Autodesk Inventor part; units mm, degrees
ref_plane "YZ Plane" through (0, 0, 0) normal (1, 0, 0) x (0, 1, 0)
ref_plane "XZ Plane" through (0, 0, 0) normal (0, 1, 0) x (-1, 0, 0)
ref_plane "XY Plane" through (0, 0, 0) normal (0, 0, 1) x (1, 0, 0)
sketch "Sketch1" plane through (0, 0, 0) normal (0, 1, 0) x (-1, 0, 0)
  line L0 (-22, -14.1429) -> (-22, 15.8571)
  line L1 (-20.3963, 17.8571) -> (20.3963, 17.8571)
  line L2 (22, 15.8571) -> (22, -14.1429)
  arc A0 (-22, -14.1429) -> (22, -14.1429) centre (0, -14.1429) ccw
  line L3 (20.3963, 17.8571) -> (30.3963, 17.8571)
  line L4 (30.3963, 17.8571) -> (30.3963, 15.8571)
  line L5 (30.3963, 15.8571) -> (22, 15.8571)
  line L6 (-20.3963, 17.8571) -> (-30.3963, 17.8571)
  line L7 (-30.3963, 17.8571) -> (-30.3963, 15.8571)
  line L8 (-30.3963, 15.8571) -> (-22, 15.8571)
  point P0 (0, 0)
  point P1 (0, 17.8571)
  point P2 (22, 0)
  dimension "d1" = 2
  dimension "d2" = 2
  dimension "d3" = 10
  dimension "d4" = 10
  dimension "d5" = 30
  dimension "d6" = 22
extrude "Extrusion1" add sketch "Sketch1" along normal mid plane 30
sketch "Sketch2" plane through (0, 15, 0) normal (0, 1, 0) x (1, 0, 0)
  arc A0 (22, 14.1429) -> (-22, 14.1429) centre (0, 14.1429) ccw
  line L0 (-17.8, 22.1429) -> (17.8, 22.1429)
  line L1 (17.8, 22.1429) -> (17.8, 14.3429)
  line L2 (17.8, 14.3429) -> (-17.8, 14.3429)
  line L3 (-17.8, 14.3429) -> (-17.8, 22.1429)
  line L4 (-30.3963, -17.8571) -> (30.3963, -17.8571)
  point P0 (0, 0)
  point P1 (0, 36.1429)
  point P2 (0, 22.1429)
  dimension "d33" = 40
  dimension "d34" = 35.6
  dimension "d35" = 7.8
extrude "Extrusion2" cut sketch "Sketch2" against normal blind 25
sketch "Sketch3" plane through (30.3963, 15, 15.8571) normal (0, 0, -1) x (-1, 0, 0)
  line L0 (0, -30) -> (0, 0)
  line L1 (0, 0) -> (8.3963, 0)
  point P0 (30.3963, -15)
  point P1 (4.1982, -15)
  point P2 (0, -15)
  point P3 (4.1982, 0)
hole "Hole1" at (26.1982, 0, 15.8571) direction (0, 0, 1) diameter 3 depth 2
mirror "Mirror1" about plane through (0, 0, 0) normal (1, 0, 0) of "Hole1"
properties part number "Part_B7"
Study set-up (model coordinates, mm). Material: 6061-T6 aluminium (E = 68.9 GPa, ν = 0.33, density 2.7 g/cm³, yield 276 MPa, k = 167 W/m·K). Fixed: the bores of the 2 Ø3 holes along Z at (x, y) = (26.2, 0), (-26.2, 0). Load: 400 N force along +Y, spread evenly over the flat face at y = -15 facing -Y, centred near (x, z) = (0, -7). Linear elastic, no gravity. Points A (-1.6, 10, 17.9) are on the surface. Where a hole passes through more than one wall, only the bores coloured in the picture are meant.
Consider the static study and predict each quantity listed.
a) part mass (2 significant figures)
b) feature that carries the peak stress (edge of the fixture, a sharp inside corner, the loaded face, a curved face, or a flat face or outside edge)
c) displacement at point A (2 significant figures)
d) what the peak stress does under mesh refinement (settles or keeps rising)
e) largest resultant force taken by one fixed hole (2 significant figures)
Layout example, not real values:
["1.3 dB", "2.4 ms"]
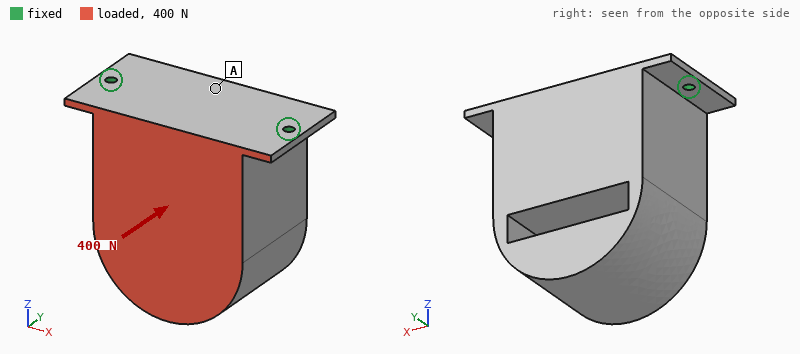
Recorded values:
["160 g", "edge of the fixture", "0.12 mm", "keeps rising", "200 N"]
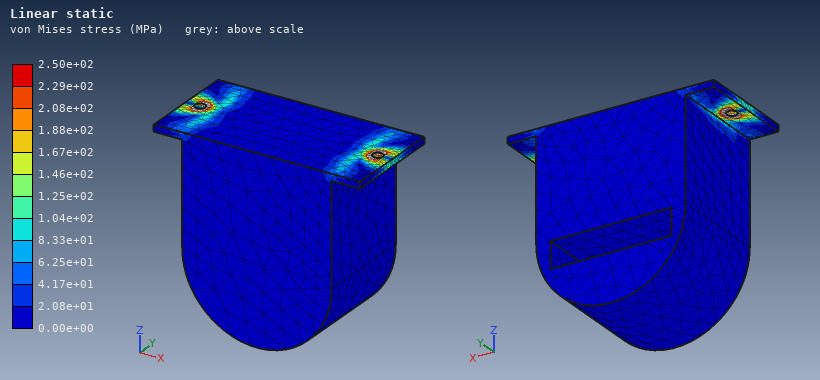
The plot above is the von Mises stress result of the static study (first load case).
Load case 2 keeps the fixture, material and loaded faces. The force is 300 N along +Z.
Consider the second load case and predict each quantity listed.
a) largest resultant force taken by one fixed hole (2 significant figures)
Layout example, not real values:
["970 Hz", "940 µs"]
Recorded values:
["170 N"]
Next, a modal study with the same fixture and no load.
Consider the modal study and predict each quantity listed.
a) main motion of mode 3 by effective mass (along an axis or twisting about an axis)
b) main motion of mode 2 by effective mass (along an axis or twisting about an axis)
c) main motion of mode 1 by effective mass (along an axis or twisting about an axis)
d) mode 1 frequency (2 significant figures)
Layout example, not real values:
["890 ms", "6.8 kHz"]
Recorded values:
["along Z", "along X", "along Y", "390 Hz"]
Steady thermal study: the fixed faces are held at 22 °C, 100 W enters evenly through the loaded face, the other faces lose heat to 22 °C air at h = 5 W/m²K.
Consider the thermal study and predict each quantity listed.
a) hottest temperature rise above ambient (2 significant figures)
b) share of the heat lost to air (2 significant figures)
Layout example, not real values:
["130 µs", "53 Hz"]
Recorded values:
["78 K", "3.5 %"]
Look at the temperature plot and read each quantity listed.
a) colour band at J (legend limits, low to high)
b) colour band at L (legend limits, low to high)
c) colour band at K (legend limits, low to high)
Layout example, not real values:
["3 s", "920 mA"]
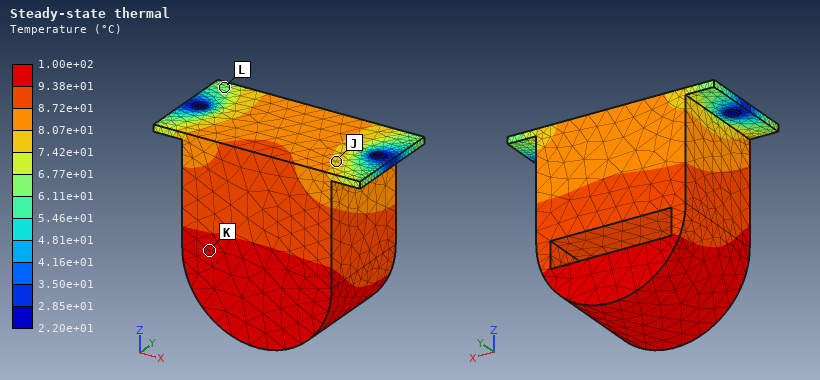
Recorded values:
["7.42e+01 to 8.07e+01 °C", "6.11e+01 to 6.77e+01 °C", "9.38e+01 to 1.00e+02 °C"]
